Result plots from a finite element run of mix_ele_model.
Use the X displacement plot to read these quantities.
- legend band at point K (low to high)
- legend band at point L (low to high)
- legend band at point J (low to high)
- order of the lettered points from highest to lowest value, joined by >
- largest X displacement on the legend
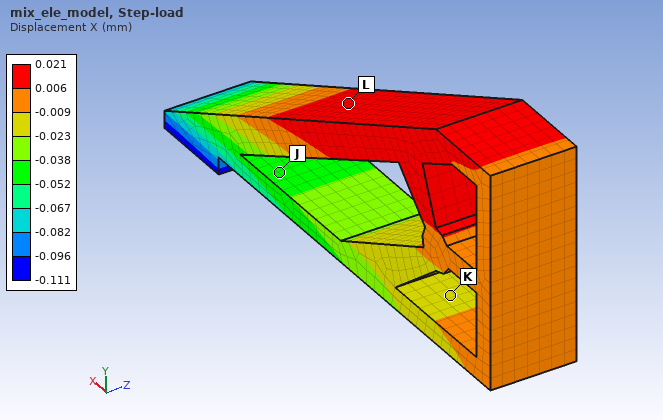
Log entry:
-0.023 to -0.009 mm
0.006 to 0.021 mm
-0.052 to -0.038 mm
L > K > J
0.021 mm
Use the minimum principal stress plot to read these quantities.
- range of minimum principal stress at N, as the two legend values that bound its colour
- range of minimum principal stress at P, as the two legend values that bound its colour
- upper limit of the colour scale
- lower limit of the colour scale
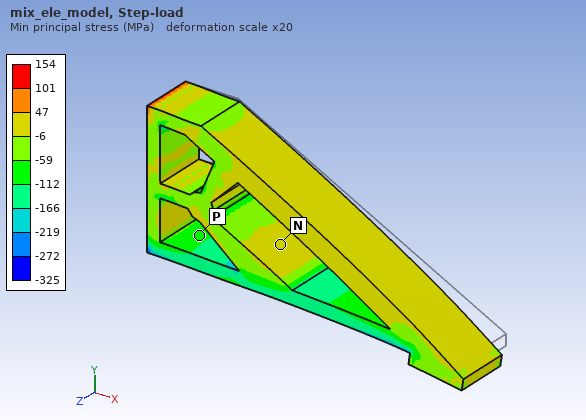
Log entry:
-6 to 47 MPa
-112 to -59 MPa
154 MPa
-325 MPa
